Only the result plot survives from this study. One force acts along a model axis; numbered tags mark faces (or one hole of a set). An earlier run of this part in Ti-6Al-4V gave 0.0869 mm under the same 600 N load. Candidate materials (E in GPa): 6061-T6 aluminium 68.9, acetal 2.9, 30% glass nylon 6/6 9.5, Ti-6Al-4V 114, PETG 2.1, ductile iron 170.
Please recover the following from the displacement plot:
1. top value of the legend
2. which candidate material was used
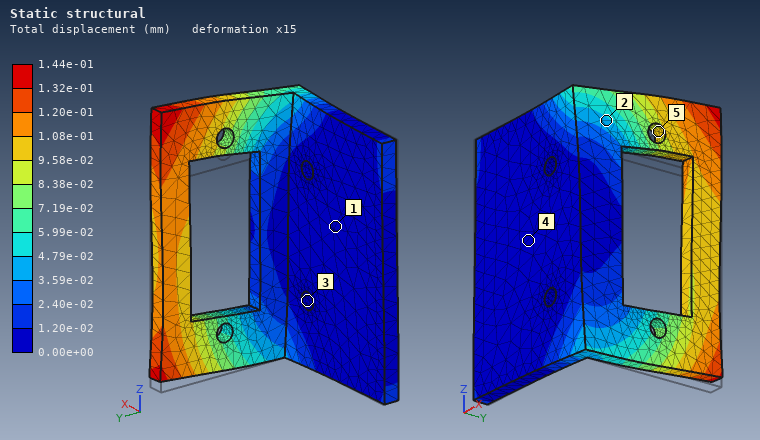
1.44e-01 mm
6061-T6 aluminium
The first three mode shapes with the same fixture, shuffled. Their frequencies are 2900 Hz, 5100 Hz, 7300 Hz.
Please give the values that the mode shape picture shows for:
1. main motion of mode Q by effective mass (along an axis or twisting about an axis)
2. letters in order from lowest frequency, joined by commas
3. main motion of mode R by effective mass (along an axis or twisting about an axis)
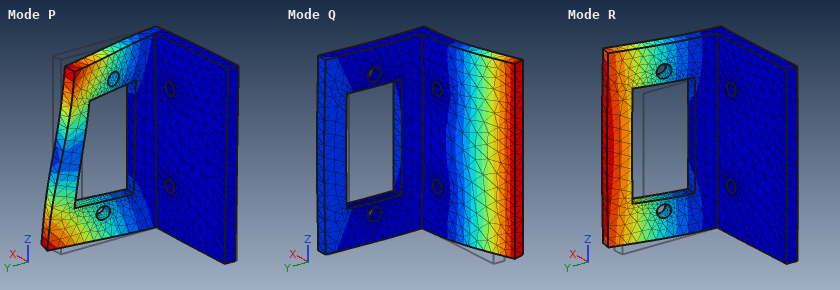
along Y
R, P, Q
along X
